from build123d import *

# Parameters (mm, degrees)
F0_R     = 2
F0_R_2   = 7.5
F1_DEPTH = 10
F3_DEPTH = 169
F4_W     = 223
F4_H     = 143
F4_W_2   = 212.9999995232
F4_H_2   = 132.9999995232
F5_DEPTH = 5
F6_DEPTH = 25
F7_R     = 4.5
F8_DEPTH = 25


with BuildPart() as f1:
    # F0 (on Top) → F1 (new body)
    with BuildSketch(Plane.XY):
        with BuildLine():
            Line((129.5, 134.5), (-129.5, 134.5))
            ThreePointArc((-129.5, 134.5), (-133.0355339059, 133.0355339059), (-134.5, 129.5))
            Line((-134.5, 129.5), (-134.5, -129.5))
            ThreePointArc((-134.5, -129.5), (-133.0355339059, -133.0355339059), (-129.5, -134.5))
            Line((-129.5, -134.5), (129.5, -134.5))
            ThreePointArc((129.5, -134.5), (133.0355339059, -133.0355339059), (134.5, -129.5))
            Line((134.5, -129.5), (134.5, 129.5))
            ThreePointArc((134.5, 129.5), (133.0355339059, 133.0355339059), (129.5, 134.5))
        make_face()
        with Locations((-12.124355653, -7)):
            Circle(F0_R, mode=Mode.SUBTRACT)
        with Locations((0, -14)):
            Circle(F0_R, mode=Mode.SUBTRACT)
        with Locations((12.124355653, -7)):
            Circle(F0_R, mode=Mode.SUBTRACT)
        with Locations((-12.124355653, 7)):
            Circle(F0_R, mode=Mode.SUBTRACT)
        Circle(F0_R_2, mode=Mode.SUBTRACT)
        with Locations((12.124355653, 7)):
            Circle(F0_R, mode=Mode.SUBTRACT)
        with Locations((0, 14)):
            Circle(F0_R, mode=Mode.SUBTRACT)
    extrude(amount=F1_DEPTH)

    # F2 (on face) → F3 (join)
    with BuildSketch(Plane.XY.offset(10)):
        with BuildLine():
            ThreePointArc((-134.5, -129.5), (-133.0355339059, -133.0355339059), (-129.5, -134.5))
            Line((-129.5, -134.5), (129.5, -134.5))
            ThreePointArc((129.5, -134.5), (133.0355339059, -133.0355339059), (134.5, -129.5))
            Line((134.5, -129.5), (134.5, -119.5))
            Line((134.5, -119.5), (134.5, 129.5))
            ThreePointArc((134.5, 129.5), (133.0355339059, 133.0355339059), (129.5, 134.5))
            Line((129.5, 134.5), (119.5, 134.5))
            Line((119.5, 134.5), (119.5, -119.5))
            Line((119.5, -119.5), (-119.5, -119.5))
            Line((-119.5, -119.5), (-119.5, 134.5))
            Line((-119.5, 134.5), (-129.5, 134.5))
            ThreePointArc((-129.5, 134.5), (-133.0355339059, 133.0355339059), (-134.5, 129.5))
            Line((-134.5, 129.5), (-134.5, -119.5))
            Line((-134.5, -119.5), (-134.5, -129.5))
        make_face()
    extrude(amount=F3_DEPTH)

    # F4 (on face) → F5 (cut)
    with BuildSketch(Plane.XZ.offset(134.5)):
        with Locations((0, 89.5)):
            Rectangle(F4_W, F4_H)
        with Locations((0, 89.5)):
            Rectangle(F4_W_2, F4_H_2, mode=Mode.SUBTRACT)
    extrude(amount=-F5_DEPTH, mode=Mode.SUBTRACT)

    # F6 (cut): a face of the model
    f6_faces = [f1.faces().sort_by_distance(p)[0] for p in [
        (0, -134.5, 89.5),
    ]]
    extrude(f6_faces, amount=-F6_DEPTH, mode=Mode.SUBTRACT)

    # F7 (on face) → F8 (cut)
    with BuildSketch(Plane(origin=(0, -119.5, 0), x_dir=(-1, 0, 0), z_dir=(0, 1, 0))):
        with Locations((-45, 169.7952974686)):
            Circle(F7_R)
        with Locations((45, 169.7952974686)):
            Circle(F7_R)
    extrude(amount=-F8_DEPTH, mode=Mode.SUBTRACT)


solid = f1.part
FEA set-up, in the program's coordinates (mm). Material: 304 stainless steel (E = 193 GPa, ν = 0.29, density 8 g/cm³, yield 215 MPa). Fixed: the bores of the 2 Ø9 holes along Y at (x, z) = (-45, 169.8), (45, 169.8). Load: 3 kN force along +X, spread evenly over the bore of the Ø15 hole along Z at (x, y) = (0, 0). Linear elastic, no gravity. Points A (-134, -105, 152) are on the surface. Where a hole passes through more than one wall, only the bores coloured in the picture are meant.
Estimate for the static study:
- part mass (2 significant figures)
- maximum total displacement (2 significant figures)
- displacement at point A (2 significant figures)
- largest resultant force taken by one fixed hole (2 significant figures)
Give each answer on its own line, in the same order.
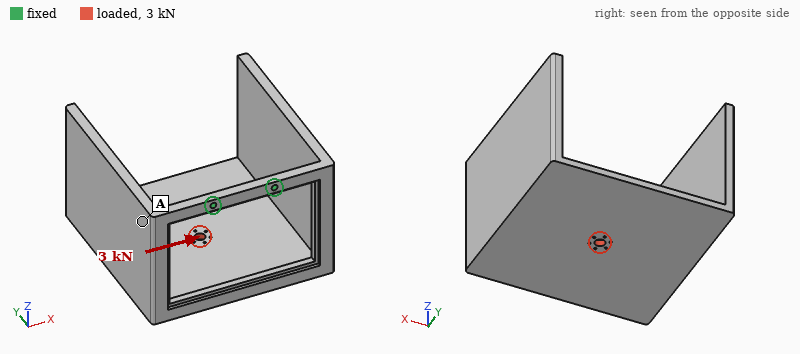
18 kg
1.3 mm
0.33 mm
3.6 kN
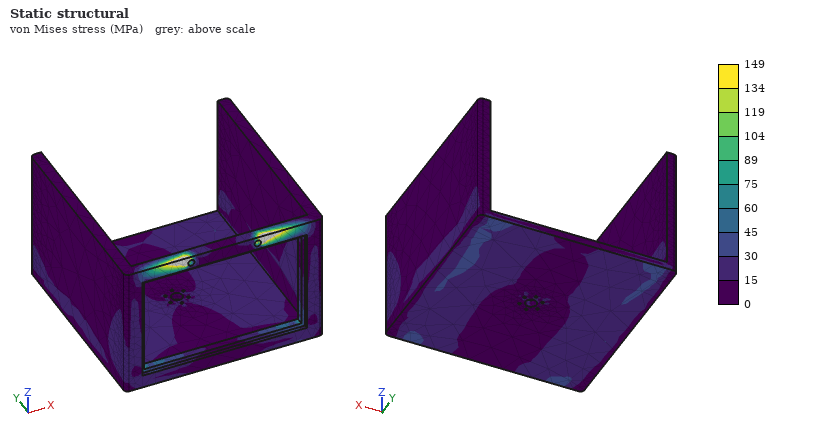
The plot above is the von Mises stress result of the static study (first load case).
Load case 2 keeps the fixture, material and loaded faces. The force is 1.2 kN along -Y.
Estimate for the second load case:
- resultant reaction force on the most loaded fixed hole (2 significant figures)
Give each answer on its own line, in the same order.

600 N
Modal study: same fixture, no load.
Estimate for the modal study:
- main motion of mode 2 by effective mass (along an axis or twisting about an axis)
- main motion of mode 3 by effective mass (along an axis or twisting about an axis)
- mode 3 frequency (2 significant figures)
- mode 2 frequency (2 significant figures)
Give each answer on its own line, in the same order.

along X
along X
120 Hz
64 Hz
